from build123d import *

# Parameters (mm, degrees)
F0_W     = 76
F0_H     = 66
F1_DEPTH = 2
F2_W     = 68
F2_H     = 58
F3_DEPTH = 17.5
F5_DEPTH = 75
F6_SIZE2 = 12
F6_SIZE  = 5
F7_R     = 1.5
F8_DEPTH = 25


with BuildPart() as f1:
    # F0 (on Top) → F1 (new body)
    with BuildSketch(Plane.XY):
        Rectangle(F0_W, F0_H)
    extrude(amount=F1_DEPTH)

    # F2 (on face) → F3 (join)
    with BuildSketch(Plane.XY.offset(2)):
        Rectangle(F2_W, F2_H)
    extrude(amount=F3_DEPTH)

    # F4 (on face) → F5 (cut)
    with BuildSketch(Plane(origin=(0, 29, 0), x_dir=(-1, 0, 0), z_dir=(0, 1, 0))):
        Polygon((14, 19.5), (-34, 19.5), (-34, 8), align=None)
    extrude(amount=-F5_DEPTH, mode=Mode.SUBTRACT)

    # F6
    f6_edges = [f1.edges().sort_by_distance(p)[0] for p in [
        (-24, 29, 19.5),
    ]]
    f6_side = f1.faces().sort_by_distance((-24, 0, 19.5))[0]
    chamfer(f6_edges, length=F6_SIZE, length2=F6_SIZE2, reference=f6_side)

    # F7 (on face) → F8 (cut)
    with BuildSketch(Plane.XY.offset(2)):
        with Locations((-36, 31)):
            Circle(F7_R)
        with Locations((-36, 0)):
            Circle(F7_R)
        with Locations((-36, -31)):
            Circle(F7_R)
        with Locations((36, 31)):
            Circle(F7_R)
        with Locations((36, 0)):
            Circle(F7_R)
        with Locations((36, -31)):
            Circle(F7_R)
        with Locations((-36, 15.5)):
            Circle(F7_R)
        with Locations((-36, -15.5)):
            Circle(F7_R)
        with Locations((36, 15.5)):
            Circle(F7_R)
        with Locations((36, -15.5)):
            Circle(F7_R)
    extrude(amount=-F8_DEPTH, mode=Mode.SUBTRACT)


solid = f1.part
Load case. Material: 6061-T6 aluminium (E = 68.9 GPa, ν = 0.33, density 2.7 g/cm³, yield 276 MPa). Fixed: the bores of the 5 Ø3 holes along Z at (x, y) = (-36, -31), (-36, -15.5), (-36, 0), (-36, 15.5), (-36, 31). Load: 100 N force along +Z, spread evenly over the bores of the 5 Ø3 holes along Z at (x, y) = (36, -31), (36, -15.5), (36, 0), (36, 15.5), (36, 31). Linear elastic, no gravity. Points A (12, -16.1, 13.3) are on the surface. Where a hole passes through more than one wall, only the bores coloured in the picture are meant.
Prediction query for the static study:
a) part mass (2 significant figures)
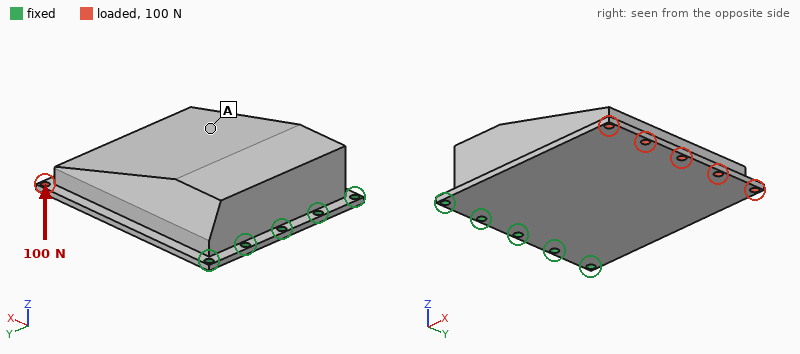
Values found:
170 g
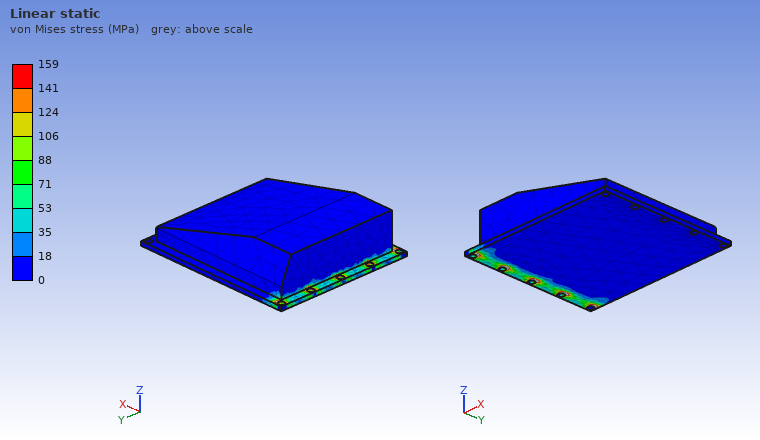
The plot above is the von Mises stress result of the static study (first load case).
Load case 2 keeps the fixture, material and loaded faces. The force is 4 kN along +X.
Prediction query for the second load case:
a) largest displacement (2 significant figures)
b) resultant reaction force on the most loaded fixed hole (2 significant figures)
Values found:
97 µm
970 N
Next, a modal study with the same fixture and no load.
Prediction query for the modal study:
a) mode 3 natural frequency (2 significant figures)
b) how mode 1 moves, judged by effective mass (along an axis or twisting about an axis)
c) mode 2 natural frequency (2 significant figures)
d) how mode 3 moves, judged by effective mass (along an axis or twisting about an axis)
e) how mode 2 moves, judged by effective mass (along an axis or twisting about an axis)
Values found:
5200 Hz
along Z
4100 Hz
along Y
along Y
